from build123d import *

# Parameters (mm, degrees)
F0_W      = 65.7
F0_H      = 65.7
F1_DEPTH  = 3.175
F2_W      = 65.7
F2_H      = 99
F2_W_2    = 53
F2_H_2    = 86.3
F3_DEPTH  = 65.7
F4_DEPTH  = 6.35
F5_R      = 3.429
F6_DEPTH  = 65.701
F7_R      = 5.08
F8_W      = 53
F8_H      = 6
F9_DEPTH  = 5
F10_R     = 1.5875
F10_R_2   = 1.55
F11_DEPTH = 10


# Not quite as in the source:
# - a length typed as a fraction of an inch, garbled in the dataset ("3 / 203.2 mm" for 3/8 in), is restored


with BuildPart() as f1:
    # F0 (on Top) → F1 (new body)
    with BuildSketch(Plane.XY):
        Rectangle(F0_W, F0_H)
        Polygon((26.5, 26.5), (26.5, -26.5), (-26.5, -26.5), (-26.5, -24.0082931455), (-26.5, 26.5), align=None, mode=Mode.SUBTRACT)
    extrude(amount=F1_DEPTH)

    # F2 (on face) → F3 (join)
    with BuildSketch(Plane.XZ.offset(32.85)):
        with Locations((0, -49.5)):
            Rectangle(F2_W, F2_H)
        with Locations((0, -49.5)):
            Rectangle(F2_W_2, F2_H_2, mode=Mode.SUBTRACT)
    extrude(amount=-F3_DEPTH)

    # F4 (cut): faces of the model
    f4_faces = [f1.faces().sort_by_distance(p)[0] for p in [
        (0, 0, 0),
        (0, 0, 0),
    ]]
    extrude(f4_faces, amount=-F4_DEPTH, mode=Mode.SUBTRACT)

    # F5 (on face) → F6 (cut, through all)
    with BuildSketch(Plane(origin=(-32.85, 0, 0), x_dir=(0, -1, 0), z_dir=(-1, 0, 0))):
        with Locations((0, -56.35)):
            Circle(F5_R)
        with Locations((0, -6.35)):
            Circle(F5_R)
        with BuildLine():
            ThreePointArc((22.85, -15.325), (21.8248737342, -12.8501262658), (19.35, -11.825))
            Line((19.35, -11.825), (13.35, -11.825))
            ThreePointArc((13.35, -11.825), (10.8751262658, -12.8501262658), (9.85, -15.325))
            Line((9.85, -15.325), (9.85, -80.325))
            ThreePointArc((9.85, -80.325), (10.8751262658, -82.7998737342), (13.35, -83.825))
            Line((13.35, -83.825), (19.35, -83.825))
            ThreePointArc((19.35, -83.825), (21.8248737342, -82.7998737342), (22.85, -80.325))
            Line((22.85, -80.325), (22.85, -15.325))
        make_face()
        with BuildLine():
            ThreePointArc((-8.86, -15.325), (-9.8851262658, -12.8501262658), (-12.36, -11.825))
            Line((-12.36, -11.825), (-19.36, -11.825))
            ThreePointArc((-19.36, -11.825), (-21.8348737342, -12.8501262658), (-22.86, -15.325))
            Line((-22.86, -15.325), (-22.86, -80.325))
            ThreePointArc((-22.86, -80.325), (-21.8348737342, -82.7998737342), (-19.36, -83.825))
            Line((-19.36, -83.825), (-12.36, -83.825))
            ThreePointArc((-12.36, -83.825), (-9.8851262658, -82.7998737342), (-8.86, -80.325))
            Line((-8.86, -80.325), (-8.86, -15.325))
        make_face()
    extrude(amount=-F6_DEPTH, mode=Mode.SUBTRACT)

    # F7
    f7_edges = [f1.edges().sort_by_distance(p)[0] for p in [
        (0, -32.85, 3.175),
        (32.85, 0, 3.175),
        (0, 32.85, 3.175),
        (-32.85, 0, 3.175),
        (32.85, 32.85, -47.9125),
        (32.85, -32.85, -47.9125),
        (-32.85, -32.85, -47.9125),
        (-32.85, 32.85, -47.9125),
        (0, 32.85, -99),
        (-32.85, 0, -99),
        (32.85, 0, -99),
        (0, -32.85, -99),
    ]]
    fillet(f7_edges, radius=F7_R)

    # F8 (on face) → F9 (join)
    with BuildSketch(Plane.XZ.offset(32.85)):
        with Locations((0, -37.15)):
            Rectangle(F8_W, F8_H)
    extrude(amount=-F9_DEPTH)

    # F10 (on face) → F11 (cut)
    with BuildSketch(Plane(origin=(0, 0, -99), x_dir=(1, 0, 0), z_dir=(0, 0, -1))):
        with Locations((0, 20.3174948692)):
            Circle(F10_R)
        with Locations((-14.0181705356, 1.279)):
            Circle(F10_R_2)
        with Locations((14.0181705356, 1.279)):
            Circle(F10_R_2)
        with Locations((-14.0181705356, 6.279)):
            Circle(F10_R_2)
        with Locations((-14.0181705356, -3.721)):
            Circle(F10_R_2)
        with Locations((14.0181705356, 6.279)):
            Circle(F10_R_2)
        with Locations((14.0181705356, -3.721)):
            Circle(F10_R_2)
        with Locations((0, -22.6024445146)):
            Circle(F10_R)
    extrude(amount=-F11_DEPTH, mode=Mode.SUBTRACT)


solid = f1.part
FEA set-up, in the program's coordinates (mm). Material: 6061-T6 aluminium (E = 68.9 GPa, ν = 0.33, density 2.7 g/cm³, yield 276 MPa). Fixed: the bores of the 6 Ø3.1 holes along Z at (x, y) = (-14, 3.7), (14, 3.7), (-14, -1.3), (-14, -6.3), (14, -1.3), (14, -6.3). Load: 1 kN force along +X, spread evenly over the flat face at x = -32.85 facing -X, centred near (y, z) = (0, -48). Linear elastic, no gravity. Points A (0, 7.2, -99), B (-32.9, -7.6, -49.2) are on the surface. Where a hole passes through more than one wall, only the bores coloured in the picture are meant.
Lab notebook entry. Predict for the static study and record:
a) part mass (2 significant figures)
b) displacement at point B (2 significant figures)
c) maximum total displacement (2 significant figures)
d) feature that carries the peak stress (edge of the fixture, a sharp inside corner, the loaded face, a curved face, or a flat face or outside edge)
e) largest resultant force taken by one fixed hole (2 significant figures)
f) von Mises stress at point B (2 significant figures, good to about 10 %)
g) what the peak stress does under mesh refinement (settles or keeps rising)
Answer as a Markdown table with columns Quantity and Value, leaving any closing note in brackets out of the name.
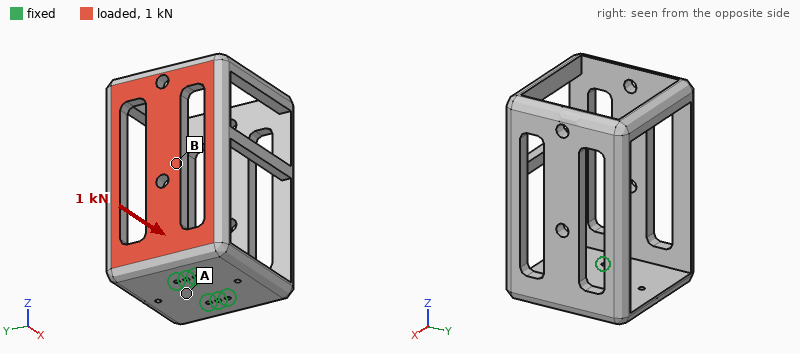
| Quantity | Value |
|---|---|
| part mass | 230 g |
| displacement at point B | 0.30 mm |
| maximum total displacement | 0.54 mm |
| feature that carries the peak stress | edge of the fixture |
| largest resultant force taken by one fixed hole | 500 N |
| von Mises stress at point B | 15 MPa |
| what the peak stress does under mesh refinement | keeps rising |
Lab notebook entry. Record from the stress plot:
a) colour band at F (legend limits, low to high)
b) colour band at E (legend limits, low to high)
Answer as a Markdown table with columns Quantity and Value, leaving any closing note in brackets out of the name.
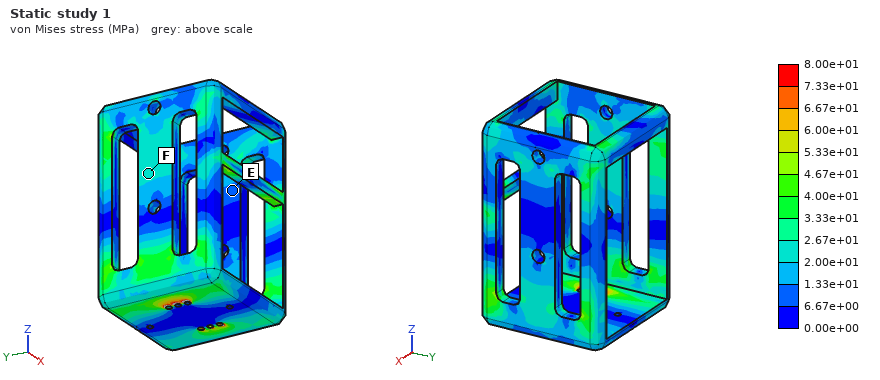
| Quantity | Value |
|---|---|
| colour band at F | 2.00e+01 to 2.67e+01 MPa |
| colour band at E | 6.67e+00 to 1.33e+01 MPa |
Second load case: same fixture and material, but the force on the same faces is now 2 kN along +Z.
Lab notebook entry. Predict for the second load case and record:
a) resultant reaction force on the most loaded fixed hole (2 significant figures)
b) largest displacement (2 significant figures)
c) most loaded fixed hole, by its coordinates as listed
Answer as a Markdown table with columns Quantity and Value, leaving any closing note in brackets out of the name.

| Quantity | Value |
|---|---|
| resultant reaction force on the most loaded fixed hole | 1.1 kN |
| largest displacement | 0.21 mm |
| most loaded fixed hole, by its coordinates as listed | (-14, 3.7) |
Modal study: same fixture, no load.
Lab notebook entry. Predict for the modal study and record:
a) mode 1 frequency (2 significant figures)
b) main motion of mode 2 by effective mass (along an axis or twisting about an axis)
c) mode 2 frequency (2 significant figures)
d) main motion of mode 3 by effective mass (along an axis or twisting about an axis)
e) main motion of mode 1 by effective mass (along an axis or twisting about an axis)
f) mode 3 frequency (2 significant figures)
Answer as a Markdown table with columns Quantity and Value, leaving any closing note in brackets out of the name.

| Quantity | Value |
|---|---|
| mode 1 frequency | 570 Hz |
| main motion of mode 2 by effective mass | along Y |
| mode 2 frequency | 790 Hz |
| main motion of mode 3 by effective mass | twisting about Z |
| main motion of mode 1 by effective mass | along X |
| mode 3 frequency | 1200 Hz |
